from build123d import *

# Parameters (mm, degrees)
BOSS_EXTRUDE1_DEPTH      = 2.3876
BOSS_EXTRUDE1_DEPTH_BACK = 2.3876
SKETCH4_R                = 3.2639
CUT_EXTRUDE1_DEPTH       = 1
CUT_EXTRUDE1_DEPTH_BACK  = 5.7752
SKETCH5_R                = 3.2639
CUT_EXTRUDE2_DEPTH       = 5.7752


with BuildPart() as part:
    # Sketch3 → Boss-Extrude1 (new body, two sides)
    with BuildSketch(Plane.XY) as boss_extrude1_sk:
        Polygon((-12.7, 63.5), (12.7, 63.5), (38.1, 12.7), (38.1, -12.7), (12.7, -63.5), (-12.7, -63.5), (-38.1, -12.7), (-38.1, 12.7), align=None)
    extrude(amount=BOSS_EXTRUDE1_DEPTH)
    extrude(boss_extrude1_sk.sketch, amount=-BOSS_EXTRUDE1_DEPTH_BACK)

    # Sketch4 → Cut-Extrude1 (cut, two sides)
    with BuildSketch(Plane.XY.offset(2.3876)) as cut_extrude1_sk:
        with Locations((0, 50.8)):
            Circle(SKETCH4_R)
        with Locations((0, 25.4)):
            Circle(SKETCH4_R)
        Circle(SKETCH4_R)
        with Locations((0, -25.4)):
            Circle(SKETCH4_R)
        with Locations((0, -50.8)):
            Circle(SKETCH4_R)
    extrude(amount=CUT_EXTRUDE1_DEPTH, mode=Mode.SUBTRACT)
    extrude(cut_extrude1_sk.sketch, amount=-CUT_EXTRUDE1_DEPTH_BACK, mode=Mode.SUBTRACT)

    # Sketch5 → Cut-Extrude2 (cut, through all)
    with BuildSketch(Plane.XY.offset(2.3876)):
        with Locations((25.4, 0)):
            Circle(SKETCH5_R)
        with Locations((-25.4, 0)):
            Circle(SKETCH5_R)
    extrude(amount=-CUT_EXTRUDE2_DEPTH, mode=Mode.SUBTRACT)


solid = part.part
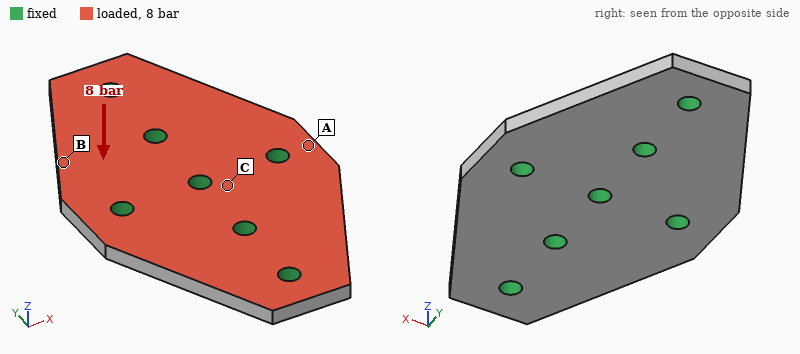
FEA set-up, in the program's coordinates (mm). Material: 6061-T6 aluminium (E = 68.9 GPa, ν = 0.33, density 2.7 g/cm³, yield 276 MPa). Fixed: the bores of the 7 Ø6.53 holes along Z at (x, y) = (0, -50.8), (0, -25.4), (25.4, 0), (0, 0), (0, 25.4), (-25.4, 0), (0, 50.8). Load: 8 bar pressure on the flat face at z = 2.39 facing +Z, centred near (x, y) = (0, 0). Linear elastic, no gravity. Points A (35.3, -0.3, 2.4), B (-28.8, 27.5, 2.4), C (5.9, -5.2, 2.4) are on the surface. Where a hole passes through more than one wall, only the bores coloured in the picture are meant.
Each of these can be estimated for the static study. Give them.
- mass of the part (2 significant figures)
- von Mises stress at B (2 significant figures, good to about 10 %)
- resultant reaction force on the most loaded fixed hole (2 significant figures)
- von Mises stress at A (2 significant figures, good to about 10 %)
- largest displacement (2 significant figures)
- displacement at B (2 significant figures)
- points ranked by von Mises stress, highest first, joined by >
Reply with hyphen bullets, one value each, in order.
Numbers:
- 88 g
- 15 MPa
- 910 N
- 27 MPa
- 36 µm
- 32 µm
- A > B > C
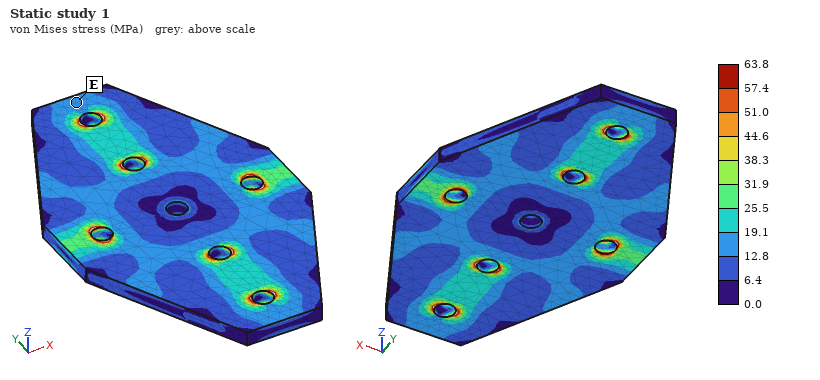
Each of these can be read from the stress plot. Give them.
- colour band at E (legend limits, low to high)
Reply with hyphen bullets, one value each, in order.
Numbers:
- 12.8 to 19.1 MPa
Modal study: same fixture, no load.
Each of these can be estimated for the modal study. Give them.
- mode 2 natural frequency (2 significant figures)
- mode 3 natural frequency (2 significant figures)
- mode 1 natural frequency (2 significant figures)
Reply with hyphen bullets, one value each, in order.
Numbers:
- 8600 Hz
- 8700 Hz
- 8300 Hz
